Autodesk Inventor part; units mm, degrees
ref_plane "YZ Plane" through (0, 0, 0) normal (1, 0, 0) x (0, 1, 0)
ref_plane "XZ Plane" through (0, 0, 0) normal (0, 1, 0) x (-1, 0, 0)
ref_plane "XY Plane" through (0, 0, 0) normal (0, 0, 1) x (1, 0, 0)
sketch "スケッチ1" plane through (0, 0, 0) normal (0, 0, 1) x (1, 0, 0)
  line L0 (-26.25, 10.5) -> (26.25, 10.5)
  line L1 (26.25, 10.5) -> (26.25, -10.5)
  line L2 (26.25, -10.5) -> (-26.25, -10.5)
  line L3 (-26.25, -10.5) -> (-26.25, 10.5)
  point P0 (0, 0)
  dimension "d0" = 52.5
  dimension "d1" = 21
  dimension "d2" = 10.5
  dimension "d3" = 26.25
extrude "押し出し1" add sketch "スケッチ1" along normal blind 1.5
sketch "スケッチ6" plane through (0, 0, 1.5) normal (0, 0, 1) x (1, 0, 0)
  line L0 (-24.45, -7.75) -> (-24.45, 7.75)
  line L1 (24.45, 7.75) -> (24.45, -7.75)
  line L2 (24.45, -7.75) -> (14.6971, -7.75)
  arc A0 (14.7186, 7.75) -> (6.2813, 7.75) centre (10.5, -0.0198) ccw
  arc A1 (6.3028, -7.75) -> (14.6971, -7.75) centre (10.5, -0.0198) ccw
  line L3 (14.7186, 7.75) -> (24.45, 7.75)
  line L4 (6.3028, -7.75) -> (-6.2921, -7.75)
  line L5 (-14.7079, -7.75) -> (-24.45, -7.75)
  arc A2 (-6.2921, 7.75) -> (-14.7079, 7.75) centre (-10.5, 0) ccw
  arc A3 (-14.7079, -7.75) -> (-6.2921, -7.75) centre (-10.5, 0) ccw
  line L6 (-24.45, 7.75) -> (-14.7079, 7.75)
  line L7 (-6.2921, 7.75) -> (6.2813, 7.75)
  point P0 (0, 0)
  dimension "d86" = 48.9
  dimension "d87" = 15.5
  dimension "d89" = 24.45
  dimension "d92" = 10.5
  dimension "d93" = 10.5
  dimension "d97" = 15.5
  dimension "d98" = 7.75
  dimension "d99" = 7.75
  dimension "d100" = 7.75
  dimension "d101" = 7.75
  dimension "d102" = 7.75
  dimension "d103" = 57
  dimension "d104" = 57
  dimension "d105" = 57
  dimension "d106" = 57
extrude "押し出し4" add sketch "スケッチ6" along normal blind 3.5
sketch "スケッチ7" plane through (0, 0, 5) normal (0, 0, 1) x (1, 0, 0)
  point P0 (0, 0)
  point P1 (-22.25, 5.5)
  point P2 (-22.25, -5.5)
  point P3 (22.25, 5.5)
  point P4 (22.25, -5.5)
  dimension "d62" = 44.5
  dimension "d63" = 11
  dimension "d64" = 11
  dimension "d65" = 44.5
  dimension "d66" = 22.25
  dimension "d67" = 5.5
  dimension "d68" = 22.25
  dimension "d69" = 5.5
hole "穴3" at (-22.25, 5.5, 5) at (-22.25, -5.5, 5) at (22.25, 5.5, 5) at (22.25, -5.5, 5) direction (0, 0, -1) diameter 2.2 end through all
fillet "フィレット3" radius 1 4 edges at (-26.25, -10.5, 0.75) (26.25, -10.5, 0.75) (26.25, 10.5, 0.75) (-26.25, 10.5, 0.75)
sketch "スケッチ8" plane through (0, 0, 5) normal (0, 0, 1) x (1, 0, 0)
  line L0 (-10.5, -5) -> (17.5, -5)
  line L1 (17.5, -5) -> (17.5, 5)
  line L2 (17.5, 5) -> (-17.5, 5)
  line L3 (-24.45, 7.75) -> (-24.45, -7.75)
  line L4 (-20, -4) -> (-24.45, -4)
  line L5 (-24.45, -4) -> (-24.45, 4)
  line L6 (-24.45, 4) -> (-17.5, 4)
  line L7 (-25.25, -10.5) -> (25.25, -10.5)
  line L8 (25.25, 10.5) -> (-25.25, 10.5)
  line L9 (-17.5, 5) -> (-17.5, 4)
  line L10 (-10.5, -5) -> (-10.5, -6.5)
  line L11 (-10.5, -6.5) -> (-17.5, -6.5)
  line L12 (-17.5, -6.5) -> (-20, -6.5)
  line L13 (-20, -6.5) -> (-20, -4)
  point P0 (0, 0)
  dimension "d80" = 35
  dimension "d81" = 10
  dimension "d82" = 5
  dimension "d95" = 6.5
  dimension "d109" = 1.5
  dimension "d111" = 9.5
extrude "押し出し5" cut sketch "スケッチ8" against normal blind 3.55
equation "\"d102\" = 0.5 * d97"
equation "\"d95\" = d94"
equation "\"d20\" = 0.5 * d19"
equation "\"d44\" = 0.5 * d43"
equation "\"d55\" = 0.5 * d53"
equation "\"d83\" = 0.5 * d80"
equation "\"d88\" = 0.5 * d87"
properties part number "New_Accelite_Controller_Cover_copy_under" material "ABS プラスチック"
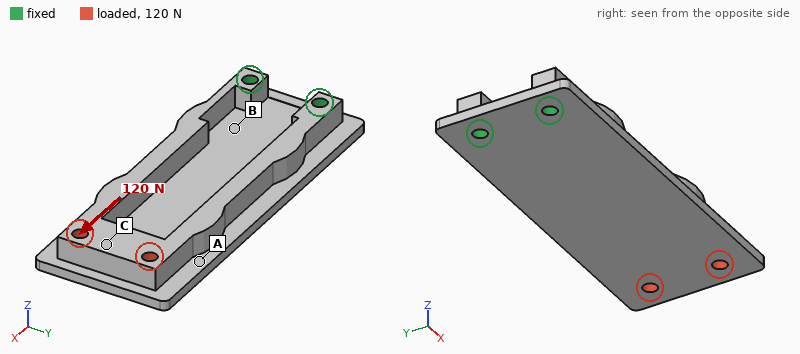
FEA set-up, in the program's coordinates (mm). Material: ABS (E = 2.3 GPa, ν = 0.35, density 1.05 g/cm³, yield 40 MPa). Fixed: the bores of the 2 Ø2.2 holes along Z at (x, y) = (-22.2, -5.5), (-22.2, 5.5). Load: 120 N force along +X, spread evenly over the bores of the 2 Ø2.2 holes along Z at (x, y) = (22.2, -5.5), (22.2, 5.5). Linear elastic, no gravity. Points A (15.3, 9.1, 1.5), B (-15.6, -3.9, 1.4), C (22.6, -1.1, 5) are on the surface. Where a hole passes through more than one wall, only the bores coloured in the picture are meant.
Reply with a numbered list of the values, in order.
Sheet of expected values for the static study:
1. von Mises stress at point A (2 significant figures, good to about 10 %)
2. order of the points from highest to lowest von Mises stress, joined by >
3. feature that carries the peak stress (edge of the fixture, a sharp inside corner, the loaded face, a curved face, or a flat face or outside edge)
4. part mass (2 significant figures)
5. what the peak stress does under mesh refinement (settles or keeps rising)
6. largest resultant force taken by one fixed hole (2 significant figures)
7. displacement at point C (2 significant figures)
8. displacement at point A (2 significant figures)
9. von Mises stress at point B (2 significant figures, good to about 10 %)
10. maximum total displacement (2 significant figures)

1. 1.9 MPa
2. B > A > C
3. a sharp inside corner
4. 3.0 g
5. keeps rising
6. 62 N
7. 0.48 mm
8. 0.30 mm
9. 3.2 MPa
10. 0.57 mm
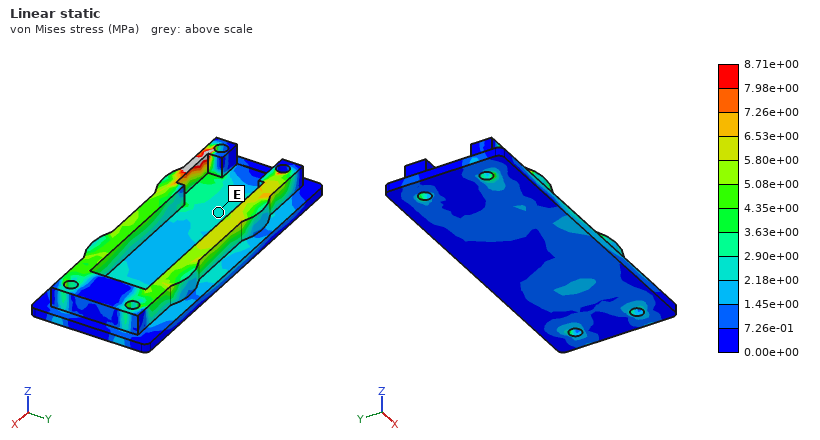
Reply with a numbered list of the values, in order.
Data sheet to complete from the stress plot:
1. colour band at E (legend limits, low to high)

1. 2.18e+00 to 2.90e+00 MPa
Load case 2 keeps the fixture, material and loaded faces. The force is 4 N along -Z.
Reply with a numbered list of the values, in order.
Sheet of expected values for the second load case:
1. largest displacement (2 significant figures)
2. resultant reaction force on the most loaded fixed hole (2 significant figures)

1. 0.68 mm
2. 4.7 N
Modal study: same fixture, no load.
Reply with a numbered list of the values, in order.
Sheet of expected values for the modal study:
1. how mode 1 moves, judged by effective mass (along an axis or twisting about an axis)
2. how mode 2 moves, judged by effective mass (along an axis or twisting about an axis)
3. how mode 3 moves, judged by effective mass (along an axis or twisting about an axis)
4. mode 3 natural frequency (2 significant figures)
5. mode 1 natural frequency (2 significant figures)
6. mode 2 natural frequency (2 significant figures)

1. along Z
2. along Y
3. along Y
4. 1700 Hz
5. 420 Hz
6. 1100 Hz
